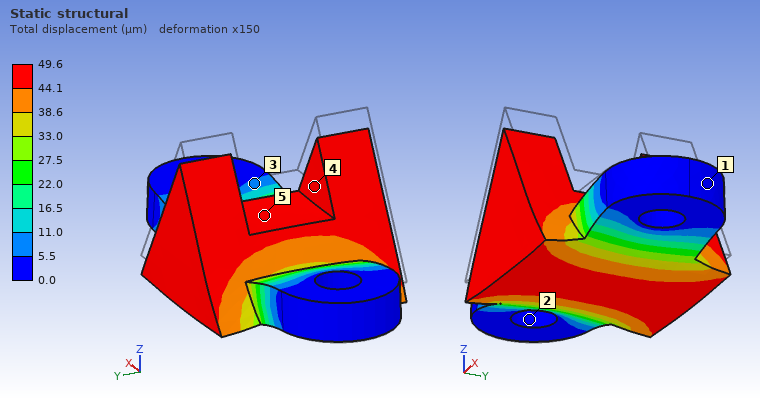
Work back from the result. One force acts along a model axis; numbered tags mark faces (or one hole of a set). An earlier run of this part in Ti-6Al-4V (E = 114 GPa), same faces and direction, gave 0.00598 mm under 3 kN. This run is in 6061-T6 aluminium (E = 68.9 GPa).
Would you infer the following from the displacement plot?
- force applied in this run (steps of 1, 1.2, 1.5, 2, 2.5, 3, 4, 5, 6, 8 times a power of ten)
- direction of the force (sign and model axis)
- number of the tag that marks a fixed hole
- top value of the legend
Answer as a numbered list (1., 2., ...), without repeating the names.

1. 15 kN
2. -Z
3. 2
4. 49.6 µm
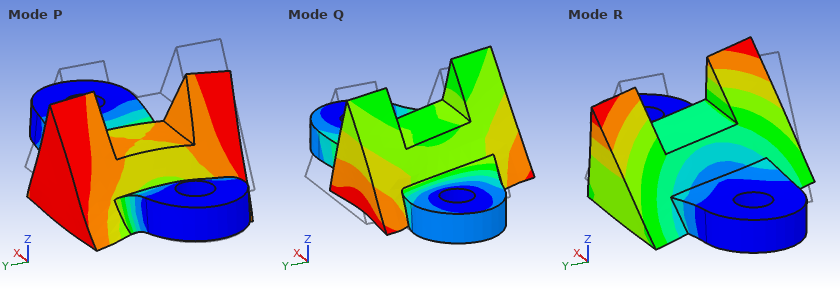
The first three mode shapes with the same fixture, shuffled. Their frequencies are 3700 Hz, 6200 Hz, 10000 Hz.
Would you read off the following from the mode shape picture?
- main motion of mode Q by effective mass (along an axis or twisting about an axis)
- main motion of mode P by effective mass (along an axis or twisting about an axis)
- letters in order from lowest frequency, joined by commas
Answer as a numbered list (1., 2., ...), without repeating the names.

1. along Y
2. along Z
3. R, P, Q
